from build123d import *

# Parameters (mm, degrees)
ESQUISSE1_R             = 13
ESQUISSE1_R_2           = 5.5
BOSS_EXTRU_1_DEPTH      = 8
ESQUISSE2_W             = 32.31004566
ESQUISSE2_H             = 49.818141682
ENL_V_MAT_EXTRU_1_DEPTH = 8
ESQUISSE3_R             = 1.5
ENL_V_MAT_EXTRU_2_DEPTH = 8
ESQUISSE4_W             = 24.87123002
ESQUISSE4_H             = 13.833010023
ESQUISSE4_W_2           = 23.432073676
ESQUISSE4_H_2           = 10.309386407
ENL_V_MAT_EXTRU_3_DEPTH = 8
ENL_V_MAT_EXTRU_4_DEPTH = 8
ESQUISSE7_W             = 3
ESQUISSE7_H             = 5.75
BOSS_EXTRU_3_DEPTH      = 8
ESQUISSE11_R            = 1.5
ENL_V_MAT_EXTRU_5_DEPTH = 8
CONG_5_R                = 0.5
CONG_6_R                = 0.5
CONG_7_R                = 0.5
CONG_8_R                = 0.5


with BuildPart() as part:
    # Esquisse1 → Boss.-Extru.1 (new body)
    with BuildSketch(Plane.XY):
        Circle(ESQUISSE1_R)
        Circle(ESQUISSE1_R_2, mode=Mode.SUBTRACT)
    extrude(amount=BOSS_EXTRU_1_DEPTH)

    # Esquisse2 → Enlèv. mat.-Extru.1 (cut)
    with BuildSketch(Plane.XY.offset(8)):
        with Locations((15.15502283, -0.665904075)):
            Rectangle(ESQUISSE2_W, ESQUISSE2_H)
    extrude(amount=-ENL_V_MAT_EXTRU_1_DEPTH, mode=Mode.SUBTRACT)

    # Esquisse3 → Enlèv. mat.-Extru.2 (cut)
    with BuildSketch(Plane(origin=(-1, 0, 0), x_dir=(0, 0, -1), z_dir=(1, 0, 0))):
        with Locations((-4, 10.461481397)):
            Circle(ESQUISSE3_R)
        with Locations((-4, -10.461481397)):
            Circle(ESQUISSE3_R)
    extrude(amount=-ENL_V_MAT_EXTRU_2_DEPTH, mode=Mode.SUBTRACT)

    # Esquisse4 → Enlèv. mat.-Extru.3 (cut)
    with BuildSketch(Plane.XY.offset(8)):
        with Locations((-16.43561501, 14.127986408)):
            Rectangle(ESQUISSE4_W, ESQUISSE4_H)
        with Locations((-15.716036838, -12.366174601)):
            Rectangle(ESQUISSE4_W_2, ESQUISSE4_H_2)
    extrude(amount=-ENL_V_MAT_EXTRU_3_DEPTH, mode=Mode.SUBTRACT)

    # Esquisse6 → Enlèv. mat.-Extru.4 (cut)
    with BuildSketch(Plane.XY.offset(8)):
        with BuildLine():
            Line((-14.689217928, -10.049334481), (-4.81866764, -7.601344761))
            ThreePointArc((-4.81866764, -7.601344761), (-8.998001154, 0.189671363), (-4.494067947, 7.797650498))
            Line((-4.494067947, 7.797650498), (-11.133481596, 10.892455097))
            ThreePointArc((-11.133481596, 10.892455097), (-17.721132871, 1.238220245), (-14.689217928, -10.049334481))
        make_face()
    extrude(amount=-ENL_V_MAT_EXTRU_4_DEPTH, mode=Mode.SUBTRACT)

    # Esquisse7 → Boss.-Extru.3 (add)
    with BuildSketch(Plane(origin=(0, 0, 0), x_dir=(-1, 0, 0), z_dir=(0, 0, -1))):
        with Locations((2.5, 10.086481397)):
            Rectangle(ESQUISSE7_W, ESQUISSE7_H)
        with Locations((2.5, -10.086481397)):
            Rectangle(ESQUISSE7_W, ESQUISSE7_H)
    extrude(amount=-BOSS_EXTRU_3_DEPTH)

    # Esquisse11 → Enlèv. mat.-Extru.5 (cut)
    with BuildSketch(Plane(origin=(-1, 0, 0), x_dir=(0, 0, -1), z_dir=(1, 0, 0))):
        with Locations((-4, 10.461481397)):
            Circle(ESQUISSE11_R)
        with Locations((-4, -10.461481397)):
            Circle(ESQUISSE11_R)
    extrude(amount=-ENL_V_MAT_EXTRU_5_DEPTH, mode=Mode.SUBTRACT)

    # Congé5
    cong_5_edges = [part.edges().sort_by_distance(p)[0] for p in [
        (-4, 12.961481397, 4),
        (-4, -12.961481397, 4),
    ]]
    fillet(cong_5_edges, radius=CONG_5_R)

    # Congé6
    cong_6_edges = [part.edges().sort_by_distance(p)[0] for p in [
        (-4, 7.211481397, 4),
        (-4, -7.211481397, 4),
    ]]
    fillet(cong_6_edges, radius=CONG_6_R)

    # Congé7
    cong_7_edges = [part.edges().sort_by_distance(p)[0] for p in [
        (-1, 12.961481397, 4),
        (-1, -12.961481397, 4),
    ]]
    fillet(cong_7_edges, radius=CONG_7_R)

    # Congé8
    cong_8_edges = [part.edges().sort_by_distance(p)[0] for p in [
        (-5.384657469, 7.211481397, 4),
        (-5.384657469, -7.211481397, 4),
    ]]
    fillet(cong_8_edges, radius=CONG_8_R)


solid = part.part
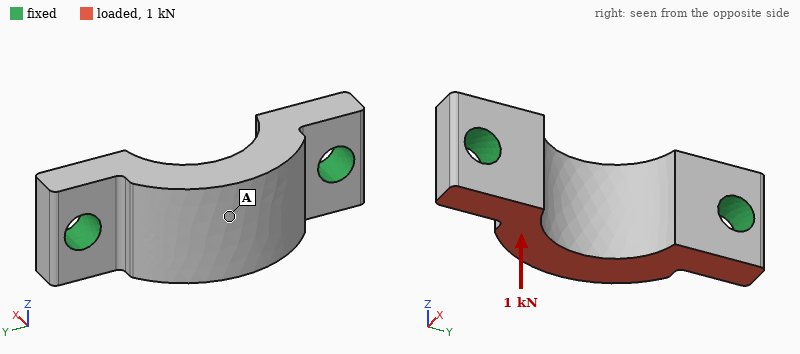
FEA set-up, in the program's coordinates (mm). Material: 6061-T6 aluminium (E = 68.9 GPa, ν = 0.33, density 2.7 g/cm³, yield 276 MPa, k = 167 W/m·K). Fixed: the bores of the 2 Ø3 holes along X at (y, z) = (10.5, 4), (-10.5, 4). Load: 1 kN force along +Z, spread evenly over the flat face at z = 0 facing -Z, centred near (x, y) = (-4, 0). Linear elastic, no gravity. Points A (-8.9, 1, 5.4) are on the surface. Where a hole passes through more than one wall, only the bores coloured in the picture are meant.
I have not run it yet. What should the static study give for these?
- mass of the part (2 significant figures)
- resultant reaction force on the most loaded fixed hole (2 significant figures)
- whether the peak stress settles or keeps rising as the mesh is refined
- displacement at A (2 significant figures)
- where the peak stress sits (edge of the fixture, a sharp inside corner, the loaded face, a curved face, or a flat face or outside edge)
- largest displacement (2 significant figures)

2.0 g
500 N
keeps rising
21 µm
edge of the fixture
24 µm
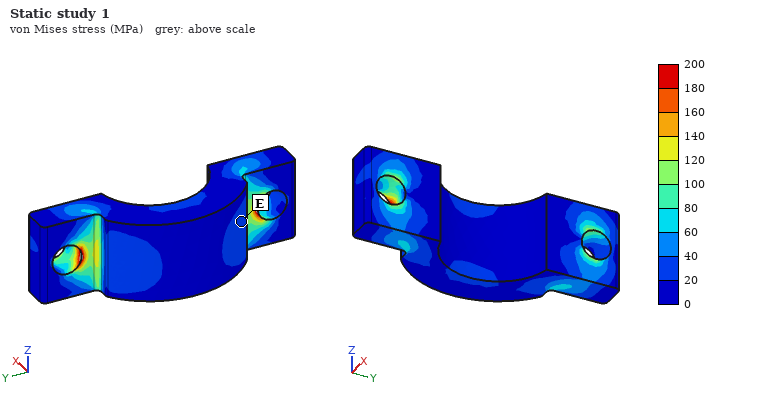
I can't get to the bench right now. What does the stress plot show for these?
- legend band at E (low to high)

20 to 40 MPa
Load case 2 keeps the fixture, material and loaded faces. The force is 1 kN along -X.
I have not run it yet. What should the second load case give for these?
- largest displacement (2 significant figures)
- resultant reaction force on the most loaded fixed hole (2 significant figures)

30 µm
560 N
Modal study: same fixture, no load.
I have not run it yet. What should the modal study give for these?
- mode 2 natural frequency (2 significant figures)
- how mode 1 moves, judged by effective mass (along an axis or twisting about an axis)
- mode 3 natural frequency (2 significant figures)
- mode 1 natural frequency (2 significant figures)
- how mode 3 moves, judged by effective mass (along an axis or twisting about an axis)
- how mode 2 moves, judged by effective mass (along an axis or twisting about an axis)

50 kHz
along Z
66 kHz
27 kHz
along Y
along X
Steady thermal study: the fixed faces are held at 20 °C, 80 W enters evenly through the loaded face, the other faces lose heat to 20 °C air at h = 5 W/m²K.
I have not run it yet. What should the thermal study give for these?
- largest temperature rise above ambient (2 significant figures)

59 K
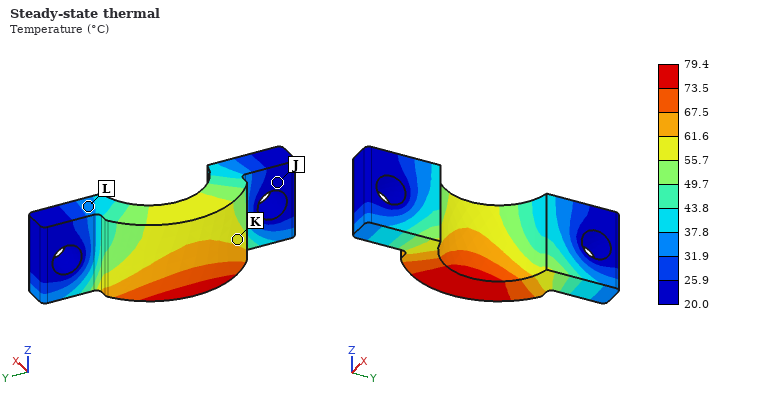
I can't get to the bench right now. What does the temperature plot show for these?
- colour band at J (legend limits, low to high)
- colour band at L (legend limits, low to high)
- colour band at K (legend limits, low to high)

20.0 to 25.9 °C
31.9 to 37.8 °C
55.7 to 61.6 °C
